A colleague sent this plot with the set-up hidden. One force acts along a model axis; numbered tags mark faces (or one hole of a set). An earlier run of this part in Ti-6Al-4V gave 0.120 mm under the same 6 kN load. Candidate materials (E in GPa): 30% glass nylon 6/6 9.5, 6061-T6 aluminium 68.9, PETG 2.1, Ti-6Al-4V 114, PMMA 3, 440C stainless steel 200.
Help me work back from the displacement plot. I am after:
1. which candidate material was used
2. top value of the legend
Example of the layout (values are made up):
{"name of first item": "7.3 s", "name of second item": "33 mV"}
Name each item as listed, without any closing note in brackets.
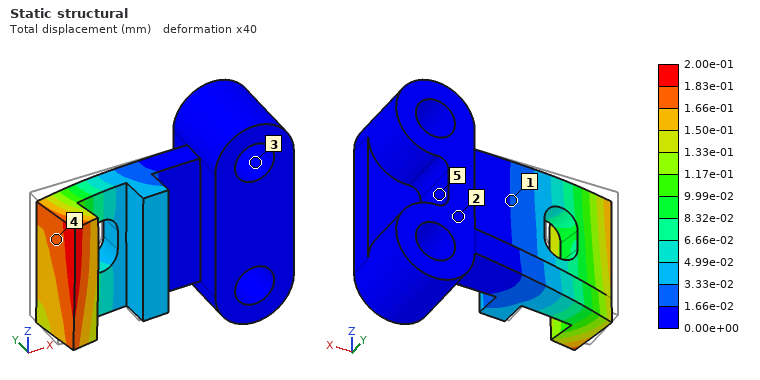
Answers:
{"which candidate material was used": "6061-T6 aluminium", "top value of the legend": "2.00e-01 mm"}
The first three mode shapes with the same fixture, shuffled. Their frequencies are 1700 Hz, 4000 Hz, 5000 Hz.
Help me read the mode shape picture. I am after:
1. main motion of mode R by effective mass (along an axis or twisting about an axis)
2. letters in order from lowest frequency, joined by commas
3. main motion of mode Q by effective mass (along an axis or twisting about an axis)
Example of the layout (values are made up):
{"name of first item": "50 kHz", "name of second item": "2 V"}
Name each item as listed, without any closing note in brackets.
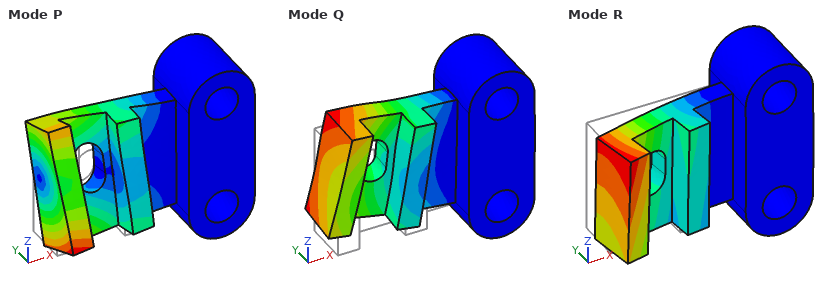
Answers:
{"main motion of mode R by effective mass": "along Y", "letters in order from lowest frequency, joined by commas": "R, P, Q", "main motion of mode Q by effective mass": "along Z"}
